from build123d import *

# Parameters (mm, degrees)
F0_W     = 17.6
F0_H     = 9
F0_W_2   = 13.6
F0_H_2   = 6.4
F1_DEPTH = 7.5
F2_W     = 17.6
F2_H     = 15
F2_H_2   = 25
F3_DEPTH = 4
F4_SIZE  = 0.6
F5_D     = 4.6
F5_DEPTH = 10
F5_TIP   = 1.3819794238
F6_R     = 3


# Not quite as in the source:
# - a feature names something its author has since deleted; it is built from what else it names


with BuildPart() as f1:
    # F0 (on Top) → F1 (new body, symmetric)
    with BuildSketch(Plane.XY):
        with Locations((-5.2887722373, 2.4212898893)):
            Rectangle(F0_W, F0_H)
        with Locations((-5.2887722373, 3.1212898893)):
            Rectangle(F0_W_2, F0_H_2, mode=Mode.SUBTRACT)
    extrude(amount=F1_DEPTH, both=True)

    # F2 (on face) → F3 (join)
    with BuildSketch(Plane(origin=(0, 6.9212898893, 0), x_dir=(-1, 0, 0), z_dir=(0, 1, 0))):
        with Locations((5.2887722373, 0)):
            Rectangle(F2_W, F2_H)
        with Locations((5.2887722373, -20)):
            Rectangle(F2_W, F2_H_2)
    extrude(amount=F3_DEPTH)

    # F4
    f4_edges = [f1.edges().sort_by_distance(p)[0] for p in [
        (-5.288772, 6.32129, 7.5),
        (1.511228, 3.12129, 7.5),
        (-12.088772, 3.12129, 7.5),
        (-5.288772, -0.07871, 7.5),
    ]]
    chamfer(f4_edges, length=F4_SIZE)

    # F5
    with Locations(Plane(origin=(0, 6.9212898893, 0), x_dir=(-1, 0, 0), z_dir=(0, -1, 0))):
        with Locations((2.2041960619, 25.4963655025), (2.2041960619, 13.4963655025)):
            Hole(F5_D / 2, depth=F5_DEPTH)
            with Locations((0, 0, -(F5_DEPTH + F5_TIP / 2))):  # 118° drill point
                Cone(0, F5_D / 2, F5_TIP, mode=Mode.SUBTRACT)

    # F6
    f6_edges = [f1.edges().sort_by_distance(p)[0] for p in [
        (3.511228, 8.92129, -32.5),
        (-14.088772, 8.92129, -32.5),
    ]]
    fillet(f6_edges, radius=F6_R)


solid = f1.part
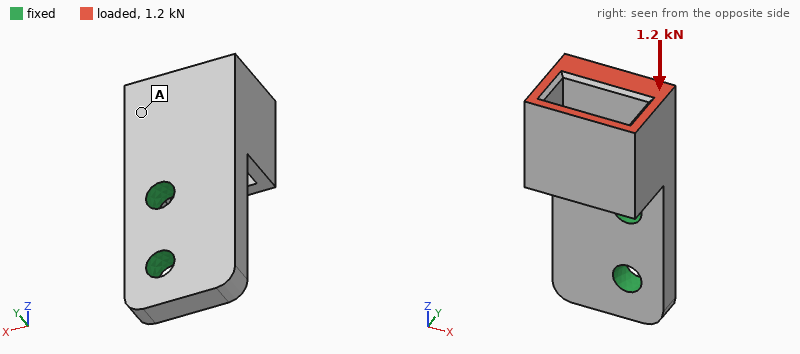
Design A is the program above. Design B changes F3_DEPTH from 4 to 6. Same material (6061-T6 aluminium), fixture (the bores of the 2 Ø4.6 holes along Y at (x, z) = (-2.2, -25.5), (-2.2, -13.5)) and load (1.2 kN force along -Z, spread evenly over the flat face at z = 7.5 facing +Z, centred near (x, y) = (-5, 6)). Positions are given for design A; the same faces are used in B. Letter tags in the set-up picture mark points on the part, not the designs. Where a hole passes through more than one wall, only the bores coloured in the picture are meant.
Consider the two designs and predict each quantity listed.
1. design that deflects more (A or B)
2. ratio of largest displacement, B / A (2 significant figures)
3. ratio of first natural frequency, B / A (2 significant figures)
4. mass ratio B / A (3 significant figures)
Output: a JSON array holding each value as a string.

["A", "0.34", "1.5", "1.36"]
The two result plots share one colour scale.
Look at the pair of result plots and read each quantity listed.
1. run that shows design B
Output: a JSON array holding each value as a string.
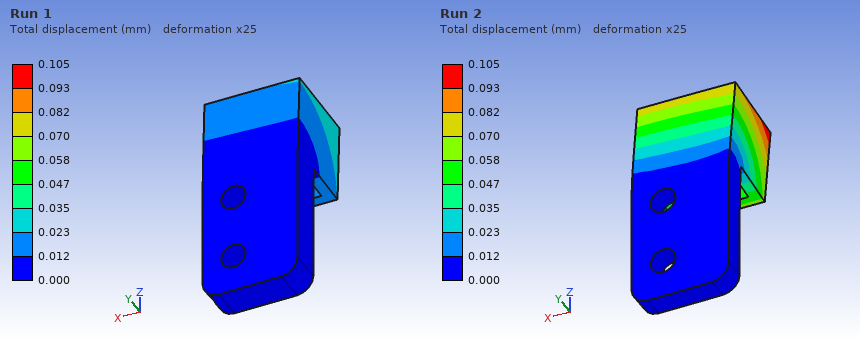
["Run 1"]
